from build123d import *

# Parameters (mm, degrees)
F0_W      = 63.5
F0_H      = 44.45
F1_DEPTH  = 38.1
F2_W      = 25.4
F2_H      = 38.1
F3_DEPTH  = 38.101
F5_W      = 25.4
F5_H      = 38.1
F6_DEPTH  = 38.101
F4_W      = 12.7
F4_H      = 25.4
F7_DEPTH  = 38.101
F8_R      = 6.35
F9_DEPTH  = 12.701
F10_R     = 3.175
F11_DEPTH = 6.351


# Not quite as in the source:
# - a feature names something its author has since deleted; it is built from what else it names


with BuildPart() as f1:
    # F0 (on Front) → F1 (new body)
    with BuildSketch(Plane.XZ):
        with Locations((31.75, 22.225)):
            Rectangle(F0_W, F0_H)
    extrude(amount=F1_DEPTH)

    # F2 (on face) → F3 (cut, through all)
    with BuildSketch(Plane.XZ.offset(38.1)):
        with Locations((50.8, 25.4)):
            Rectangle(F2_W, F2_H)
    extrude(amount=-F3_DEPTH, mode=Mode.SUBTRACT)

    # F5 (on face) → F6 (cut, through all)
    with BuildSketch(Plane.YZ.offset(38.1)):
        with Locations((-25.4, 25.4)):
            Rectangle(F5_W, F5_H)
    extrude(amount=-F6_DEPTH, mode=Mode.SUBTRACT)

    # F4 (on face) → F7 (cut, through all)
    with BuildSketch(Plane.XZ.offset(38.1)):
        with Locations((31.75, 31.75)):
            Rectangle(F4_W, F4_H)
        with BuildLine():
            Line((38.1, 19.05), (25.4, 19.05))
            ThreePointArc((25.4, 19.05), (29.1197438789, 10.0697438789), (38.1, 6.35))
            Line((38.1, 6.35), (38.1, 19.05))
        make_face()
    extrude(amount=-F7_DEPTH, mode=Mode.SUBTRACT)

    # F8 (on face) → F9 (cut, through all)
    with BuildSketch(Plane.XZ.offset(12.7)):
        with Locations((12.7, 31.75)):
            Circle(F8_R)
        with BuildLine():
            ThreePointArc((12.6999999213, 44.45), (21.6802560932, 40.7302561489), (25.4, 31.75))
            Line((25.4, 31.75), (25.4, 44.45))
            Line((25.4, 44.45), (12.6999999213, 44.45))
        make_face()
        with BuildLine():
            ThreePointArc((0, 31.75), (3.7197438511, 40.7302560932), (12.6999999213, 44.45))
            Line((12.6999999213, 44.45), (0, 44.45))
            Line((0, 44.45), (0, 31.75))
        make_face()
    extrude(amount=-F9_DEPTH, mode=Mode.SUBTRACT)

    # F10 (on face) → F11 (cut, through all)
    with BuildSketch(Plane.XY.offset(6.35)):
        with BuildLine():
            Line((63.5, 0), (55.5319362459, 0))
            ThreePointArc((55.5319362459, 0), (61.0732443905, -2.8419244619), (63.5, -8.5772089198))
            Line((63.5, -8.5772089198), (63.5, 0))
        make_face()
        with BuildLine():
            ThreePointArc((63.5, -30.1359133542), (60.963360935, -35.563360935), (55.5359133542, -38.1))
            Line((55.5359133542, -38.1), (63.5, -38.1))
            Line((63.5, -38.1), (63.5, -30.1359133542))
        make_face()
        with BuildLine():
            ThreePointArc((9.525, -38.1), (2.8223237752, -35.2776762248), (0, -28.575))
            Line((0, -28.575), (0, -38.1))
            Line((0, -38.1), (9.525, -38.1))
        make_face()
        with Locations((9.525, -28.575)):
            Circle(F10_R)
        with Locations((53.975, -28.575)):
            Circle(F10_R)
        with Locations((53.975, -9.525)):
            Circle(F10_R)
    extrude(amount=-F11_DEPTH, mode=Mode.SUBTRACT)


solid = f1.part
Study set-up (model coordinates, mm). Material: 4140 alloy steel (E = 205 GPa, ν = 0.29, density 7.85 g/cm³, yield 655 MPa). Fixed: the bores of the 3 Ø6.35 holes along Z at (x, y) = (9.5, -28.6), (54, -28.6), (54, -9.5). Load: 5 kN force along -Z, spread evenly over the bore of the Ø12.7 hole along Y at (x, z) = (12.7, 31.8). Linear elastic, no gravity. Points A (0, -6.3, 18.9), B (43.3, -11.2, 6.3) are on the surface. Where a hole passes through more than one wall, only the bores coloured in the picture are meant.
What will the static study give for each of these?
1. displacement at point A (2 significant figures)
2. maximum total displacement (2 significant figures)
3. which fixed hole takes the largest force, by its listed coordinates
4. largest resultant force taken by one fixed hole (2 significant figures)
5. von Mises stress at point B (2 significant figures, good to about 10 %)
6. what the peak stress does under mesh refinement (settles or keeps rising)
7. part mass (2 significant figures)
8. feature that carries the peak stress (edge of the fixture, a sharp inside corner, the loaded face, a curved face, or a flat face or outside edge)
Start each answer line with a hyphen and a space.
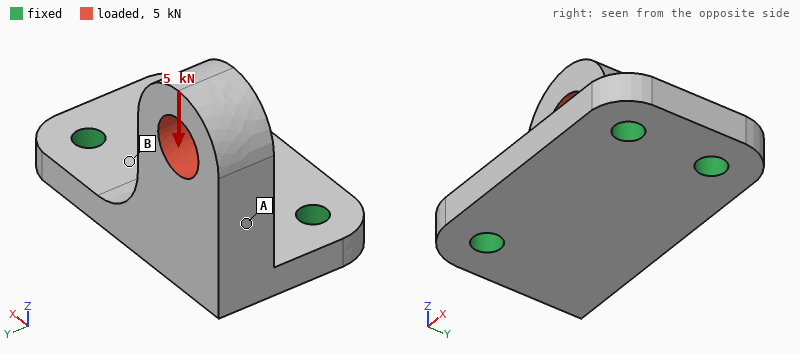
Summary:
- 0.12 mm
- 0.21 mm
- (9.5, -28.6)
- 4.0 kN
- 130 MPa
- keeps rising
- 190 g
- edge of the fixture
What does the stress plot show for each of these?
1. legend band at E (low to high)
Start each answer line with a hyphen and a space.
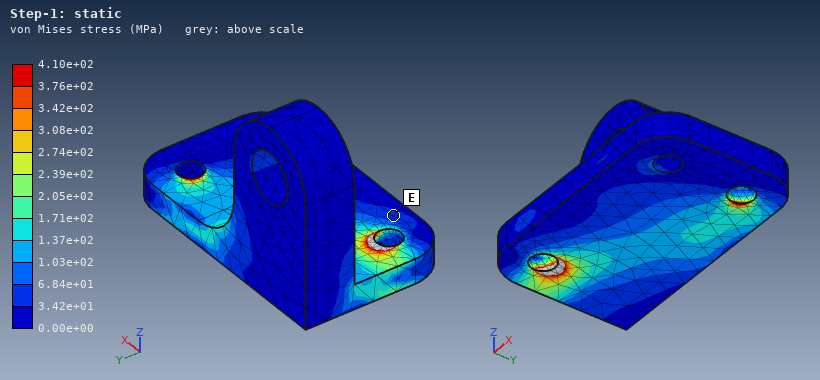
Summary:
- 3.42e+01 to 6.84e+01 MPa
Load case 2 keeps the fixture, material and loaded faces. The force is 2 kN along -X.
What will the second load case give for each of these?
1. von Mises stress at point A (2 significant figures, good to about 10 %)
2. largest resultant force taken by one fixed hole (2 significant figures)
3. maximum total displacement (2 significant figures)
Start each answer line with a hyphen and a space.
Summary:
- 23 MPa
- 1.5 kN
- 75 µm
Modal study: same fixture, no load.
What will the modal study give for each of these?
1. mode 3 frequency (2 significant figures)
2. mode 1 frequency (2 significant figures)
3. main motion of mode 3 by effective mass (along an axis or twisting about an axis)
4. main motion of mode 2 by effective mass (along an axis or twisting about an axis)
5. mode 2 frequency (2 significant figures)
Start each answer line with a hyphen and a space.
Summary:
- 7700 Hz
- 2400 Hz
- along Z
- along X
- 5100 Hz
